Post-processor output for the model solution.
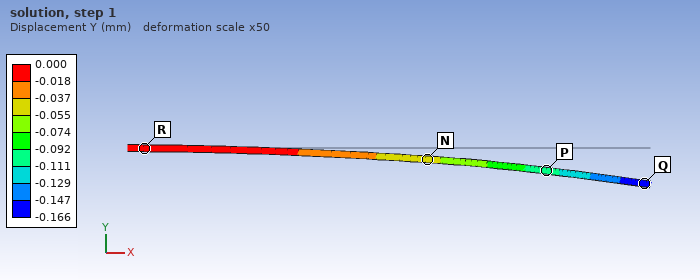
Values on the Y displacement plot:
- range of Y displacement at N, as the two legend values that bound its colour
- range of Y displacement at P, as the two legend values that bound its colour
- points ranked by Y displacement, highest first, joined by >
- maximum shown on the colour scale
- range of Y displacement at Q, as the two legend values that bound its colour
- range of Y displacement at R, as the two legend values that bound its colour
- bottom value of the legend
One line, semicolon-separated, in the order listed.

-0.055 to -0.037 mm; -0.111 to -0.092 mm; R > N > P > Q; 0.000 mm; -0.166 to -0.147 mm; -0.018 to 0.000 mm; -0.166 mm
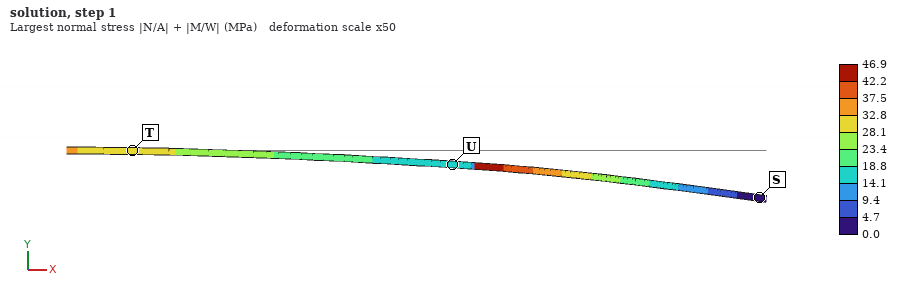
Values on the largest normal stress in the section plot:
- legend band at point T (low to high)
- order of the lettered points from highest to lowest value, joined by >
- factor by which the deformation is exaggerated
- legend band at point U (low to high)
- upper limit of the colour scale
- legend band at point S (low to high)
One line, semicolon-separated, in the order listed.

28.1 to 32.8 MPa; T > U > S; 50; 14.1 to 18.8 MPa; 46.9 MPa; 0.0 to 4.7 MPa
